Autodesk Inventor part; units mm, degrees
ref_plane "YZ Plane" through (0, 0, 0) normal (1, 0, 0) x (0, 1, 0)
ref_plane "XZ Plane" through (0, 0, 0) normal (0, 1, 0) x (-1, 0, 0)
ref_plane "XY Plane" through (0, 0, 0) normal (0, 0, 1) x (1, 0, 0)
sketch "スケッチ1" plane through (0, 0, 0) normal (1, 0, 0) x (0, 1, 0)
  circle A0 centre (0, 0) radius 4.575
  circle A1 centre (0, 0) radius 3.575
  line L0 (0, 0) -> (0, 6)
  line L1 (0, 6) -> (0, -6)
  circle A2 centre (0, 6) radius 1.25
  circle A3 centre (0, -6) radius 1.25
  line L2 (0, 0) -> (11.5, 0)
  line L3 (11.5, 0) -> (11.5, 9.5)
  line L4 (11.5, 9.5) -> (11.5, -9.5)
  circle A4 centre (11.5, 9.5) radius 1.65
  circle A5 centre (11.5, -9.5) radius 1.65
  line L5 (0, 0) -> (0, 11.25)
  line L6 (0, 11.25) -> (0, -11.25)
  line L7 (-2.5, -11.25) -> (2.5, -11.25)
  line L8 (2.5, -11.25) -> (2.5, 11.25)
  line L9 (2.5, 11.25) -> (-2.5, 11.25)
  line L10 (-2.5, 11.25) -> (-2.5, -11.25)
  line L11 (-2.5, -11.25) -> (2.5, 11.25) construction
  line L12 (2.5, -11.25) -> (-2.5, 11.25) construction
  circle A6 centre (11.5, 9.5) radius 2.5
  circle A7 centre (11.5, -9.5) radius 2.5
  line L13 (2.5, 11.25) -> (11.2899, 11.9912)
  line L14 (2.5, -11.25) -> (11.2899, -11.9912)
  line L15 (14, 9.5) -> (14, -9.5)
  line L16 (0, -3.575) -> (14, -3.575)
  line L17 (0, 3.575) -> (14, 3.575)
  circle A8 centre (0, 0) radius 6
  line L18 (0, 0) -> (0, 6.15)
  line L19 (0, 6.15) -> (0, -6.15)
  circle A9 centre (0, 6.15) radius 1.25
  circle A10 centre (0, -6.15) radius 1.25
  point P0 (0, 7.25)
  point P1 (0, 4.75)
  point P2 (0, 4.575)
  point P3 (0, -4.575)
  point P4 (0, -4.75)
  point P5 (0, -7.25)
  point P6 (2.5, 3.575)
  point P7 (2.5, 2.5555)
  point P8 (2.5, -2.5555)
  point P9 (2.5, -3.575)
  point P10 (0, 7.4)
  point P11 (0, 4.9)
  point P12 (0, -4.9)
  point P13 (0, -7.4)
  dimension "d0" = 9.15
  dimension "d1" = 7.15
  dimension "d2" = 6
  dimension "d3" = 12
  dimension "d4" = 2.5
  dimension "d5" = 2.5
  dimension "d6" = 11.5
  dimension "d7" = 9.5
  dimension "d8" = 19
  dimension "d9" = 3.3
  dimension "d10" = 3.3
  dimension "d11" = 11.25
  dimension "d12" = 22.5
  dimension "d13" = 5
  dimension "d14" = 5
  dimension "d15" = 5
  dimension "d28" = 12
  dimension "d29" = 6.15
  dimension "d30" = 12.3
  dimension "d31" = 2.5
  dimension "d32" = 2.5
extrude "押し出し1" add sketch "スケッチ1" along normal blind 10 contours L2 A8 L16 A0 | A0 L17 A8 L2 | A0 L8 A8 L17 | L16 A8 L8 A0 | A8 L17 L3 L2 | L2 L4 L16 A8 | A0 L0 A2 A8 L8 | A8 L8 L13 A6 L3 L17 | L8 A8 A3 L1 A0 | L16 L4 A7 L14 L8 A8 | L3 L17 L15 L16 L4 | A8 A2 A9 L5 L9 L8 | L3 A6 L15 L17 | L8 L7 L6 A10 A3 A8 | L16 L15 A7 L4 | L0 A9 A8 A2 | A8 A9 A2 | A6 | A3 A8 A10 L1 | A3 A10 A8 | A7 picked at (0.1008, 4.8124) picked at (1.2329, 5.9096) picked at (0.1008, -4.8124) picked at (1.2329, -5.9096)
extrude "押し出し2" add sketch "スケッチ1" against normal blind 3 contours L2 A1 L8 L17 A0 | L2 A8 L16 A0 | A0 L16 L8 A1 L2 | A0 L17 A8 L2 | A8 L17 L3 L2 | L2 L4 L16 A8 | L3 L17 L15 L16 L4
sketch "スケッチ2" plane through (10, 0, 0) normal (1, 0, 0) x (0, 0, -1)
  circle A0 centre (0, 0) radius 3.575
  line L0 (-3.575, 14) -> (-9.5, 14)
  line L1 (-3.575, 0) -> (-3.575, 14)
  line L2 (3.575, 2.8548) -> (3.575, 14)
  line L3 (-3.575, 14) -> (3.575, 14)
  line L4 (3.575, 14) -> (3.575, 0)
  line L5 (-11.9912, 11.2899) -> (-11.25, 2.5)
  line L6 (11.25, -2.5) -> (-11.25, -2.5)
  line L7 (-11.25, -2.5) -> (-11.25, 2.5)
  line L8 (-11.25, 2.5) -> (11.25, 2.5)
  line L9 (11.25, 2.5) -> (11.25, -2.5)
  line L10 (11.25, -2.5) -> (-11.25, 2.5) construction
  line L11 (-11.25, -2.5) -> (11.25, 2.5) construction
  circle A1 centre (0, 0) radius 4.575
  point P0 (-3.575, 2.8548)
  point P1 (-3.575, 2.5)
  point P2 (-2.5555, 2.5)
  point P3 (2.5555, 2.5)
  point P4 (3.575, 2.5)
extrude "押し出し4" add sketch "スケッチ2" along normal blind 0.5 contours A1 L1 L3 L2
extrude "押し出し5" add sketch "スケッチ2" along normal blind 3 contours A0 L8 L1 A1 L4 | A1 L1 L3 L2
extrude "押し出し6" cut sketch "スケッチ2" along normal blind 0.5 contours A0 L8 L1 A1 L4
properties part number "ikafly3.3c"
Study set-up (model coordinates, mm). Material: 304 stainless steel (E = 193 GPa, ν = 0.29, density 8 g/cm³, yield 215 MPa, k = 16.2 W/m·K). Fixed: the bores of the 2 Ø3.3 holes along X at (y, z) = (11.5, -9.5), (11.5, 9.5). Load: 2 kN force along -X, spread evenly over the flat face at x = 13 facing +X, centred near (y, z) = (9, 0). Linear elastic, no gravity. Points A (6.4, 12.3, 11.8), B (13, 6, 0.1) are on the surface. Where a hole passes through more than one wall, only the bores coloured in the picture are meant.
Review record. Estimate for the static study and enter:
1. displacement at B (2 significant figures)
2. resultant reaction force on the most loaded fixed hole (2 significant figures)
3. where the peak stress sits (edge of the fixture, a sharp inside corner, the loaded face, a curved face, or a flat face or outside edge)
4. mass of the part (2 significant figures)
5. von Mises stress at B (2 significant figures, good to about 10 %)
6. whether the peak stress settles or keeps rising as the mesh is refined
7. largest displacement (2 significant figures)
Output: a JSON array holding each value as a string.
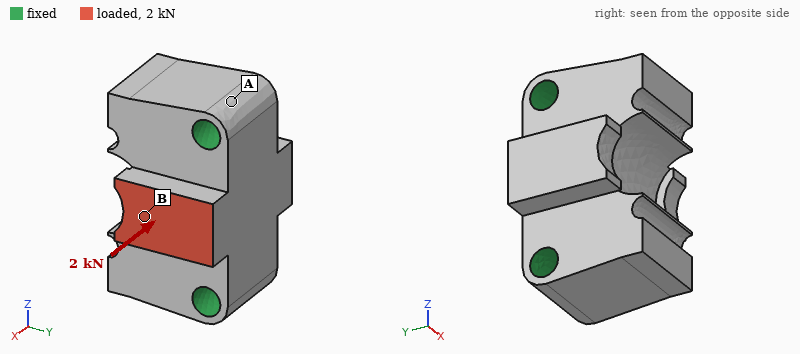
["2.5 µm", "1.0 kN", "a sharp inside corner", "25 g", "30 MPa", "keeps rising", "3.2 µm"]
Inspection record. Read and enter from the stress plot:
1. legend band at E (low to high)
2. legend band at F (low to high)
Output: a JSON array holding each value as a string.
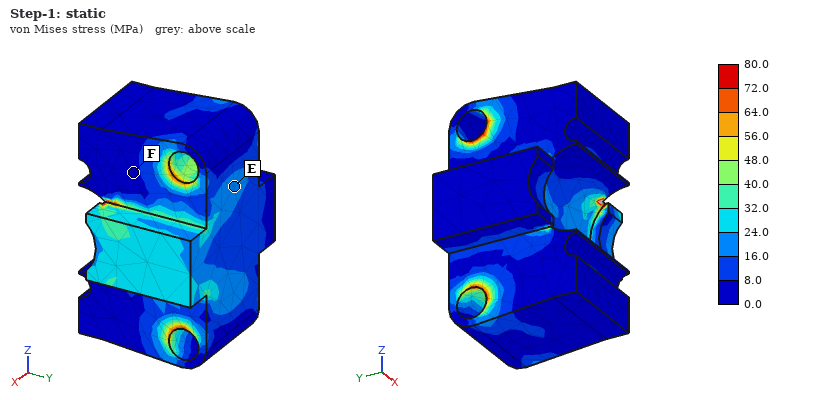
["16.0 to 24.0 MPa", "0.0 to 8.0 MPa"]
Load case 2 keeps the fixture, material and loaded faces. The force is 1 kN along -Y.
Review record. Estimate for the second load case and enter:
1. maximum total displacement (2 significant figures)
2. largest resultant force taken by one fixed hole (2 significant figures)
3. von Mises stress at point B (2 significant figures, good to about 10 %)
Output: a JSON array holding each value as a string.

["5.5 µm", "580 N", "31 MPa"]
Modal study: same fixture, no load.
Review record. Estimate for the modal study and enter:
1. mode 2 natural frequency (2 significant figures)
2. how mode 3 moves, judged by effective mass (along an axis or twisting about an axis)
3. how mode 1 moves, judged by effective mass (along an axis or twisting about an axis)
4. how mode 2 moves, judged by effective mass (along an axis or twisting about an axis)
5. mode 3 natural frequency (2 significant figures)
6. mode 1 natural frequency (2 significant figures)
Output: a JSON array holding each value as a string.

["46 kHz", "twisting about Y", "along X", "along Y", "57 kHz", "37 kHz"]
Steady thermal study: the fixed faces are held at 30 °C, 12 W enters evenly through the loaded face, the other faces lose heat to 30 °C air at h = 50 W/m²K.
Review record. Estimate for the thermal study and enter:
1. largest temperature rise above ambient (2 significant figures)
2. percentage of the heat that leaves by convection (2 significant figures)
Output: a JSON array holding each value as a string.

["77 K", "9.9 %"]
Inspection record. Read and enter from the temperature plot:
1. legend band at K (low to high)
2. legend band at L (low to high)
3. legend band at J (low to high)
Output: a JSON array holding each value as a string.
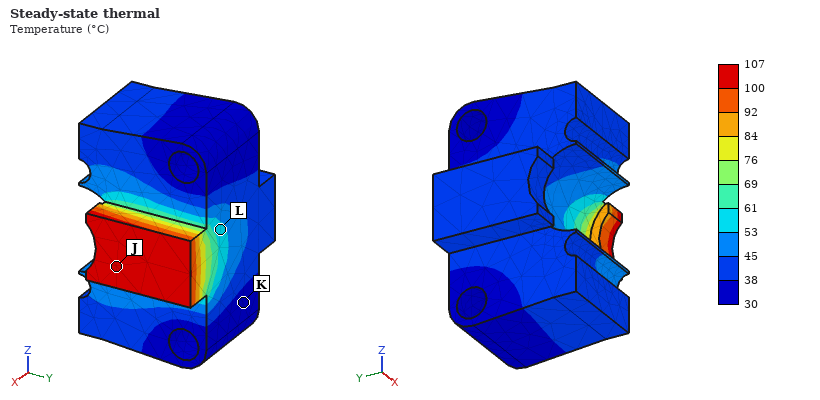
["30 to 38 °C", "53 to 61 °C", "100 to 107 °C"]
